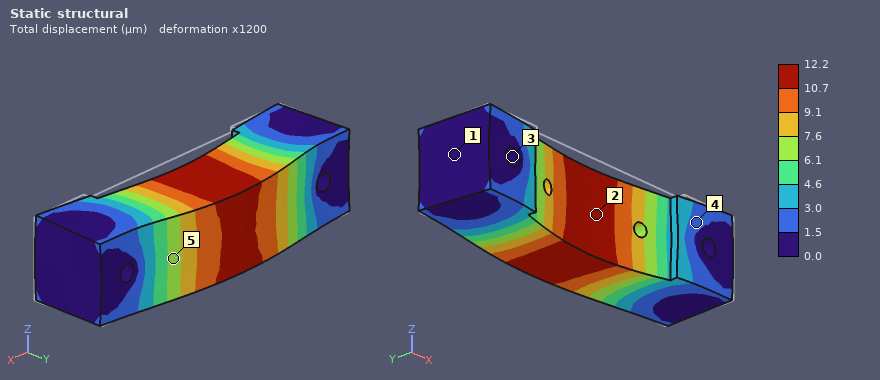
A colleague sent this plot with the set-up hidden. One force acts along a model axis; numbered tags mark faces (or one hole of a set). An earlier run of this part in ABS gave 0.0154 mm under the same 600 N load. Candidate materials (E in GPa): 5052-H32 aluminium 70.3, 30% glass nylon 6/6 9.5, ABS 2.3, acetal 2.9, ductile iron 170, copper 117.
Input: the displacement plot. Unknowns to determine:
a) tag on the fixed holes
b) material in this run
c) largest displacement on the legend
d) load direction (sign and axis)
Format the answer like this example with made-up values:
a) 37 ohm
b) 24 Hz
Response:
a) 3
b) acetal
c) 12.2 µm
d) +Y
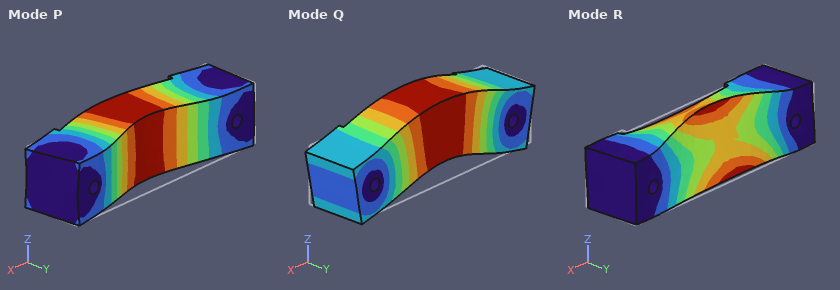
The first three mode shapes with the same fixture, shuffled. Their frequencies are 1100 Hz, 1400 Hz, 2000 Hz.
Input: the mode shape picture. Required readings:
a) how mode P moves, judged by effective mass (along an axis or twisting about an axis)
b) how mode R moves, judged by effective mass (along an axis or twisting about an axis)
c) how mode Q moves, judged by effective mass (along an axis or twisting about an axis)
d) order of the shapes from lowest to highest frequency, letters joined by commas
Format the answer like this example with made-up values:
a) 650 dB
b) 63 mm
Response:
a) along Y
b) twisting about X
c) along Z
d) Q, P, R
